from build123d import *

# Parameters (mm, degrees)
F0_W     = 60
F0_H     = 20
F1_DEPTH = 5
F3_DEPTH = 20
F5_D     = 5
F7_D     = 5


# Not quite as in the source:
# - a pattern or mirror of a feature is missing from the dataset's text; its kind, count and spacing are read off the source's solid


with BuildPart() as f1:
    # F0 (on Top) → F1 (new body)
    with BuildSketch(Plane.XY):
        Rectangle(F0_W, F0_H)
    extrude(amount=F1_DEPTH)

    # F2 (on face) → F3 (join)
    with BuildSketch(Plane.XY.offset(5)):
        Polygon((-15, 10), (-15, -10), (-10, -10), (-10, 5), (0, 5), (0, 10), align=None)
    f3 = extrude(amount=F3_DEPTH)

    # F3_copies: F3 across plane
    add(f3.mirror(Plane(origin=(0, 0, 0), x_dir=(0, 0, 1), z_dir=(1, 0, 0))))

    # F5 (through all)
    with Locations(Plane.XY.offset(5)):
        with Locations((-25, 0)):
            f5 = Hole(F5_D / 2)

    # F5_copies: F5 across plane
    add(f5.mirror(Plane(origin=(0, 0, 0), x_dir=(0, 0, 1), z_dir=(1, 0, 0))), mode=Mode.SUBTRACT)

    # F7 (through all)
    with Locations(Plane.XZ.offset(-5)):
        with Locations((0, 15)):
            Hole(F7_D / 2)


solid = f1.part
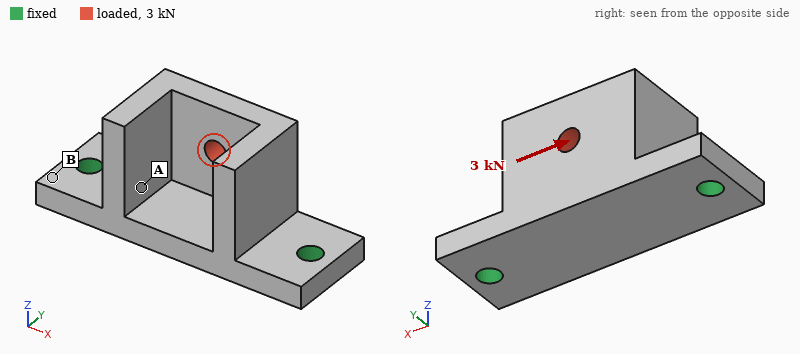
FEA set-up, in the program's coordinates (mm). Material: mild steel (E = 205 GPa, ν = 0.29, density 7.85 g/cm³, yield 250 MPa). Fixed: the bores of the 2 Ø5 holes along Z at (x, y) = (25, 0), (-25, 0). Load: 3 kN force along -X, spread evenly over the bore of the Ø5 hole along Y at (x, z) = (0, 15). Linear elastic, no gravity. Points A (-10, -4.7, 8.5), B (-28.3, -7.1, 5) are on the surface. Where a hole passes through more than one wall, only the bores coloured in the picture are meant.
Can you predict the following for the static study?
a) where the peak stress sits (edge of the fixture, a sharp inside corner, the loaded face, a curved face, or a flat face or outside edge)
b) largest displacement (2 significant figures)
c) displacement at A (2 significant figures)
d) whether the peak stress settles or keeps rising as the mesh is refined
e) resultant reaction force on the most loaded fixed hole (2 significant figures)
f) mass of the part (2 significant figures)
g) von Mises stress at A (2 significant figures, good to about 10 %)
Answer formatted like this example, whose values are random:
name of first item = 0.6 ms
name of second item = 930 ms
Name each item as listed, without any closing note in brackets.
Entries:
where the peak stress sits = edge of the fixture
largest displacement = 15 µm
displacement at A = 2.7 µm
whether the peak stress settles or keeps rising as the mesh is refined = keeps rising
resultant reaction force on the most loaded fixed hole = 1.8 kN
mass of the part = 92 g
von Mises stress at A = 23 MPa
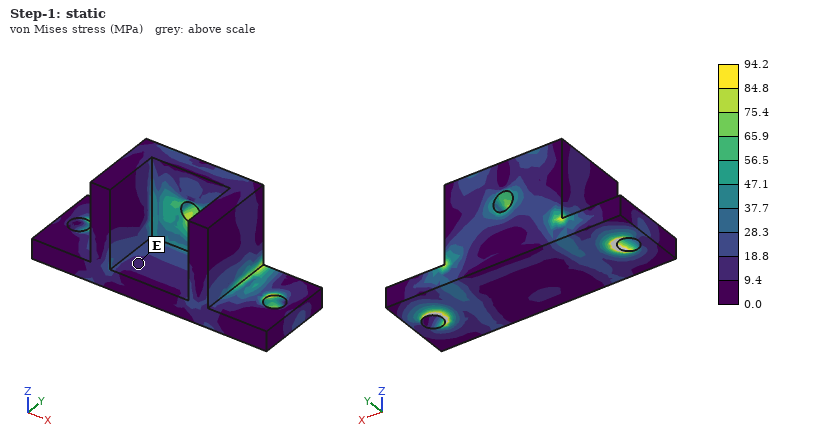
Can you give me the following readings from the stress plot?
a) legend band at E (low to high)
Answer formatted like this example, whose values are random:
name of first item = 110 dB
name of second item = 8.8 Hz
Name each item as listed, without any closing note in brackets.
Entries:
legend band at E = 9.4 to 18.8 MPa
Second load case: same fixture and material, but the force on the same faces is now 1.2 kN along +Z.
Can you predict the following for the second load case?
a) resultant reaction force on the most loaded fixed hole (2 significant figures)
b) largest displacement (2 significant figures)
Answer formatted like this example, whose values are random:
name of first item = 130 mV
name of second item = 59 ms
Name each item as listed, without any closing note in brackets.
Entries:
resultant reaction force on the most loaded fixed hole = 650 N
largest displacement = 20 µm
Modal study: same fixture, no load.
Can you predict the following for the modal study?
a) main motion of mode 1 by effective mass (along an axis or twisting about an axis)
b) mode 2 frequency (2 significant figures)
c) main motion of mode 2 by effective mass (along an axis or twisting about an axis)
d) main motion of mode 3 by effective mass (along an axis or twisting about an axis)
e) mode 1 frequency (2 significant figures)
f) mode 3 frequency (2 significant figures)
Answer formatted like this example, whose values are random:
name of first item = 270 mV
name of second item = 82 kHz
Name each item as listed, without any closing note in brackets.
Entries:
main motion of mode 1 by effective mass = along Y
mode 2 frequency = 9500 Hz
main motion of mode 2 by effective mass = along Z
main motion of mode 3 by effective mass = along X
mode 1 frequency = 5000 Hz
mode 3 frequency = 9900 Hz
